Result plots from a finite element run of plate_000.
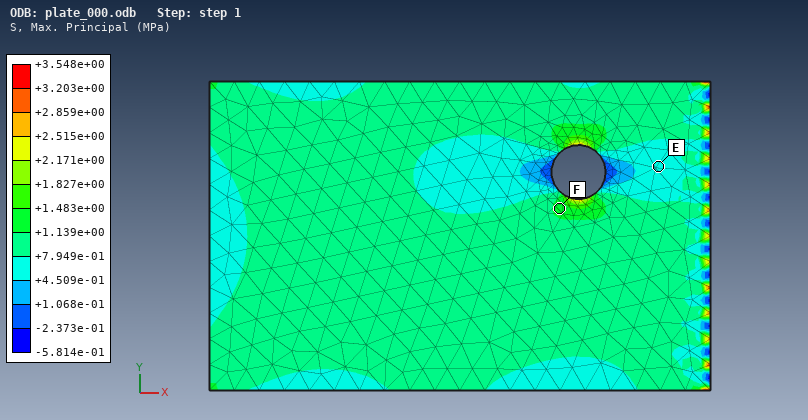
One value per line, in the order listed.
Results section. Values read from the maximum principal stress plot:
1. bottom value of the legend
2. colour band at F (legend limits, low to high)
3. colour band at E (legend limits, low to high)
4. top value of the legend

-5.814e-01 MPa
+1.139e+00 to +1.483e+00 MPa
+4.509e-01 to +7.949e-01 MPa
+3.548e+00 MPa
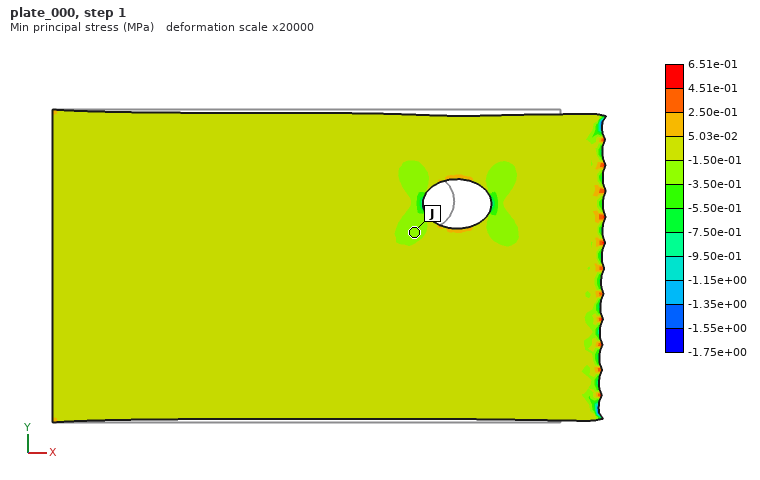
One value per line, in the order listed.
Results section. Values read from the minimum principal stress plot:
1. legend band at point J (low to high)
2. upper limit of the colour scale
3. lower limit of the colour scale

-3.50e-01 to -1.50e-01 MPa
6.51e-01 MPa
-1.75e+00 MPa
